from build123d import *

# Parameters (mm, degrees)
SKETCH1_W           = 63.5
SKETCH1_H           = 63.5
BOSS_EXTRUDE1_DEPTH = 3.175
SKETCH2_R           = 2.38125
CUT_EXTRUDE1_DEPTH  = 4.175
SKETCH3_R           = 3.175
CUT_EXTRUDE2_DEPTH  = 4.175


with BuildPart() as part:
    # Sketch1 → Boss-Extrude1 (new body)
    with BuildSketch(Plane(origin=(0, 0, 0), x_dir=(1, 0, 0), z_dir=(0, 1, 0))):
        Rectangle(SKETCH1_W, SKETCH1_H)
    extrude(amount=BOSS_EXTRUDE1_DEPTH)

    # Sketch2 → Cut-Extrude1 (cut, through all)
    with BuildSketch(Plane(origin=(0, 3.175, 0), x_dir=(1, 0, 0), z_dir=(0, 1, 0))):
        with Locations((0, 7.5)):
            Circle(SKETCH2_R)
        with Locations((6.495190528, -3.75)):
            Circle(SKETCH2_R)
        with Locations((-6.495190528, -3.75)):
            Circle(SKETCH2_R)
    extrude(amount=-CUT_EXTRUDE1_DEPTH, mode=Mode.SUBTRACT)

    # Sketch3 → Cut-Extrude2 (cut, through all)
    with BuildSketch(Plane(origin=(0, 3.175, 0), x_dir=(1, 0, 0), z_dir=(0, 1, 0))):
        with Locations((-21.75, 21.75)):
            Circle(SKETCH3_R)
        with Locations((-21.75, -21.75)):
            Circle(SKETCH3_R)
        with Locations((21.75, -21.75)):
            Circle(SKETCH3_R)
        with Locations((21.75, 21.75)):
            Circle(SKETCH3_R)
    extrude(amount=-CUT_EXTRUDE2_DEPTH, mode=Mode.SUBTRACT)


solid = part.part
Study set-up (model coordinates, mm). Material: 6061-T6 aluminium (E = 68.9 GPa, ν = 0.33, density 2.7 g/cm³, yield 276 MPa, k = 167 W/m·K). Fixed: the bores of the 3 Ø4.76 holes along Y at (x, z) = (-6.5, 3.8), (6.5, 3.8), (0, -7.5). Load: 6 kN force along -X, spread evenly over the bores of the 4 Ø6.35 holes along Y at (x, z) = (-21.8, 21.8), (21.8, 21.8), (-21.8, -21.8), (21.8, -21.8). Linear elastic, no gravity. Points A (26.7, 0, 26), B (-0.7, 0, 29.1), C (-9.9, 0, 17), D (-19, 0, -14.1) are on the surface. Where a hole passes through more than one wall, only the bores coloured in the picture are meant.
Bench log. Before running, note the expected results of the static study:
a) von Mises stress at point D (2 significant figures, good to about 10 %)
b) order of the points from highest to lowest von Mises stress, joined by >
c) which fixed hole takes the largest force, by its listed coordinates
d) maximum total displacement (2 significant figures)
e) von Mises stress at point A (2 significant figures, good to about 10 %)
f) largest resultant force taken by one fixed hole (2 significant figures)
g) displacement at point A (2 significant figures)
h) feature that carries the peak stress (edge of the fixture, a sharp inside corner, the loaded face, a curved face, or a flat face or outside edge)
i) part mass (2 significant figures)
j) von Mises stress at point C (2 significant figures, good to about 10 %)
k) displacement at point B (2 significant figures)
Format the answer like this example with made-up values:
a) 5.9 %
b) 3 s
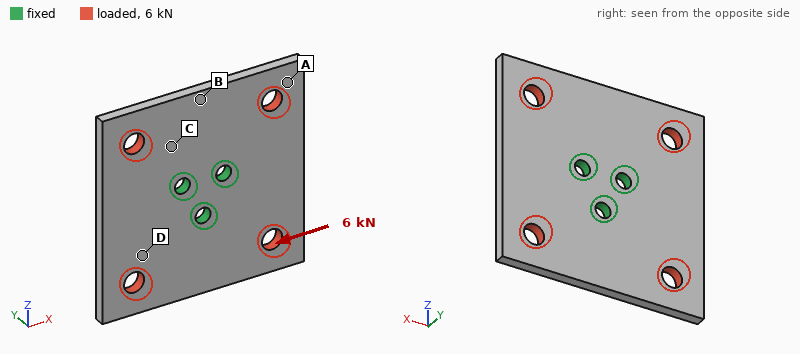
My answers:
a) 36 MPa
b) D > C > A > B
c) (0, -7.5)
d) 22 µm
e) 14 MPa
f) 2.3 kN
g) 21 µm
h) edge of the fixture
i) 33 g
j) 26 MPa
k) 17 µm
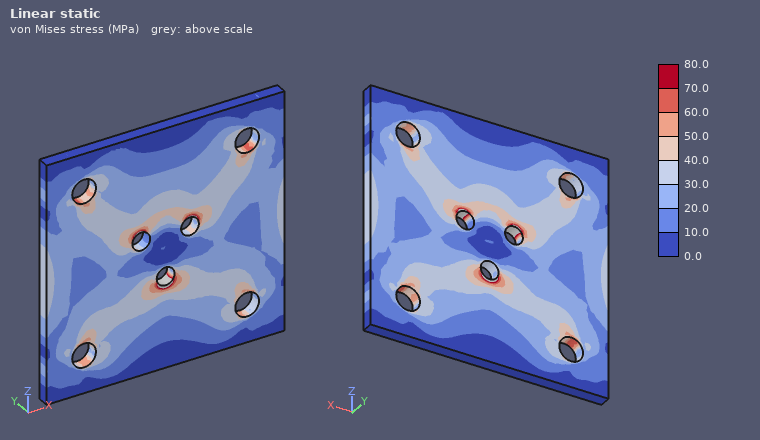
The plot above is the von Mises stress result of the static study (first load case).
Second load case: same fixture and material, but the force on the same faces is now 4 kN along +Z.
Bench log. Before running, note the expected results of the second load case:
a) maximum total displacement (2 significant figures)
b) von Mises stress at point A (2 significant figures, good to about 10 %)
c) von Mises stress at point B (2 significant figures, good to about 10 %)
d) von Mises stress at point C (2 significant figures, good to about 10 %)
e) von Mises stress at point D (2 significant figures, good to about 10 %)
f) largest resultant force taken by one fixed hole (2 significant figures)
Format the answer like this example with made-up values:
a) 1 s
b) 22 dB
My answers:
a) 14 µm
b) 9.3 MPa
c) 19 MPa
d) 20 MPa
e) 19 MPa
f) 1.5 kN
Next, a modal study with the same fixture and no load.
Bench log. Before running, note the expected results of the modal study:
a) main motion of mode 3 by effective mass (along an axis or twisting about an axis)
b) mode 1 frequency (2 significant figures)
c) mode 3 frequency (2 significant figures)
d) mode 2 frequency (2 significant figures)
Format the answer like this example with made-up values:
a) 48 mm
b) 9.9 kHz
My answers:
a) along Y
b) 2700 Hz
c) 3100 Hz
d) 2800 Hz
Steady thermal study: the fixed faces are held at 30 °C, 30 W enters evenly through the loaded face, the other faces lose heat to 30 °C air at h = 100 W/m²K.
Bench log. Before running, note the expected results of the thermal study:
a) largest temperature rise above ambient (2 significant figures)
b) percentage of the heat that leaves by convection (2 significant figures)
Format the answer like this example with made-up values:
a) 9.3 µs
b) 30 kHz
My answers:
a) 14 K
b) 23 %
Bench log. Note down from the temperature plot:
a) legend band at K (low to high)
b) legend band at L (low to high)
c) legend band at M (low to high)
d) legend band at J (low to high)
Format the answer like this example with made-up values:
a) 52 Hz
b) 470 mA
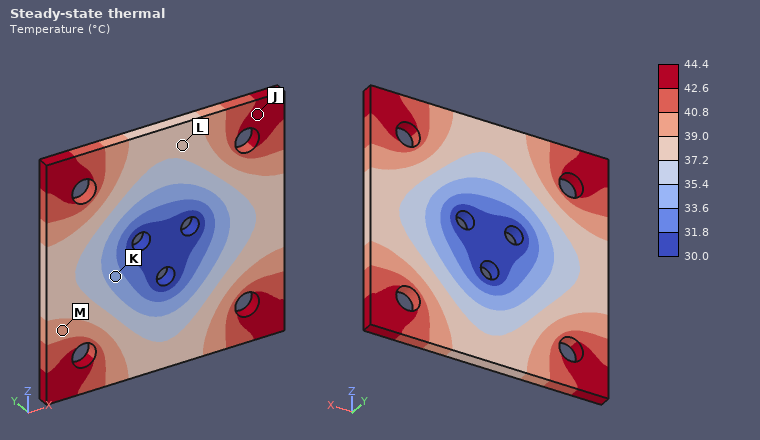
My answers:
a) 33.6 to 35.4 °C
b) 37.2 to 39.0 °C
c) 39.0 to 40.8 °C
d) 42.6 to 44.4 °C
